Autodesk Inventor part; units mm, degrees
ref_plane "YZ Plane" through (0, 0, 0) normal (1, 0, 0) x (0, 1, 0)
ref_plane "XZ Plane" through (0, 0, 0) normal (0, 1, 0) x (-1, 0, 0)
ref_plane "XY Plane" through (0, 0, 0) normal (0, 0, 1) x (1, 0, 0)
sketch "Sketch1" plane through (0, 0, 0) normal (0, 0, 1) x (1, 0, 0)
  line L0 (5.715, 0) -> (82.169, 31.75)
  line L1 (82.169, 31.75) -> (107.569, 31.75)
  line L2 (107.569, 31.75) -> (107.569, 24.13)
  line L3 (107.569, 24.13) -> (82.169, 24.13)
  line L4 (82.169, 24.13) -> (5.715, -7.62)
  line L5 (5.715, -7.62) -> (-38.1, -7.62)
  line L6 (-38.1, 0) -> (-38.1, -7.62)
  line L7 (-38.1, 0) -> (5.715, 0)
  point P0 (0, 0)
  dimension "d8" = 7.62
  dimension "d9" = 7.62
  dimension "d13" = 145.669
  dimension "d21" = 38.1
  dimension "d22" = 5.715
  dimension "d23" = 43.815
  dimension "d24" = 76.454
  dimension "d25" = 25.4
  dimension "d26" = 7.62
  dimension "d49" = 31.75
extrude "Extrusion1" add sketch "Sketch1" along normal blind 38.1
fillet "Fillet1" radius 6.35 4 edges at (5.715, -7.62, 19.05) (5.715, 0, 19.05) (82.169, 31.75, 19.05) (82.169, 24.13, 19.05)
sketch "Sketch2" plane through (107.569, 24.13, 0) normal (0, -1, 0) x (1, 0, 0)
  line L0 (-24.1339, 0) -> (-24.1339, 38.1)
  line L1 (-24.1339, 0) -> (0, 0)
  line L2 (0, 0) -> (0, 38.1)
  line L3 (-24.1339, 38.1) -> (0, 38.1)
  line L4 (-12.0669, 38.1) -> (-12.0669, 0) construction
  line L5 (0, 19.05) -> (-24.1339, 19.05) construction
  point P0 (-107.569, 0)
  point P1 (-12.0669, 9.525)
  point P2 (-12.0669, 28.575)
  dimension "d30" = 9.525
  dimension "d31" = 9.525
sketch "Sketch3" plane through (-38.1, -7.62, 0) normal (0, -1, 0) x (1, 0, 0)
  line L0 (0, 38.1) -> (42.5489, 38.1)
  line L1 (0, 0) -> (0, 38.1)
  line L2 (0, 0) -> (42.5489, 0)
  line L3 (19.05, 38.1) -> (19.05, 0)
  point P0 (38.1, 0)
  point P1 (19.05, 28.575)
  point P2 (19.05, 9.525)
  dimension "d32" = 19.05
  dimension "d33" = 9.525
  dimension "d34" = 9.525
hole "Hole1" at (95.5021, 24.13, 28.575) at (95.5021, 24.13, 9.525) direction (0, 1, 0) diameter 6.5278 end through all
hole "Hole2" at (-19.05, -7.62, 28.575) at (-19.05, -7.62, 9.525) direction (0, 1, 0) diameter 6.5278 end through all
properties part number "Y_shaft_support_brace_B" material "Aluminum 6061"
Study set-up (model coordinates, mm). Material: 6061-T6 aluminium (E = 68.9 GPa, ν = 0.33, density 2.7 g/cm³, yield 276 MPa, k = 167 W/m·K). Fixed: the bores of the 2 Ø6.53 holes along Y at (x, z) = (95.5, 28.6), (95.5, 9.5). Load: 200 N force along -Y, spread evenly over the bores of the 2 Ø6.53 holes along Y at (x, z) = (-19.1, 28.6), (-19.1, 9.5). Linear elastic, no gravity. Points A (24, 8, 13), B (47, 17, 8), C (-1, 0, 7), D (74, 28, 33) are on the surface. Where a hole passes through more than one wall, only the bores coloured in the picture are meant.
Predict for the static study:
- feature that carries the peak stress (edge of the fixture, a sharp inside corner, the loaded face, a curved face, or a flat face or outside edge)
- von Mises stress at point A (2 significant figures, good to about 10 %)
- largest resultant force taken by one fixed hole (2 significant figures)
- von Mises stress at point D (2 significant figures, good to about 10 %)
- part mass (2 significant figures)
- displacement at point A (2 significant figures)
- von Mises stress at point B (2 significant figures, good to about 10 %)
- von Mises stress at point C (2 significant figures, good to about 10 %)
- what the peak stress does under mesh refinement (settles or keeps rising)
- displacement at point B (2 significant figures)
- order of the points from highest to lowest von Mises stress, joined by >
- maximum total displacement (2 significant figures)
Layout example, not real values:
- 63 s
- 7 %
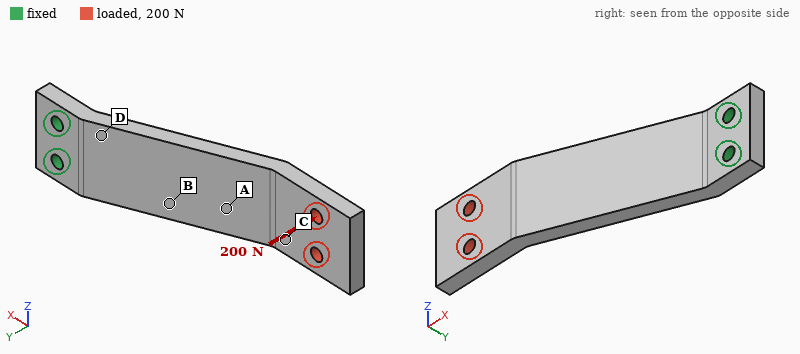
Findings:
- edge of the fixture
- 29 MPa
- 130 N
- 60 MPa
- 110 g
- 0.58 mm
- 43 MPa
- 9.9 MPa
- keeps rising
- 0.27 mm
- D > B > A > C
- 1.6 mm
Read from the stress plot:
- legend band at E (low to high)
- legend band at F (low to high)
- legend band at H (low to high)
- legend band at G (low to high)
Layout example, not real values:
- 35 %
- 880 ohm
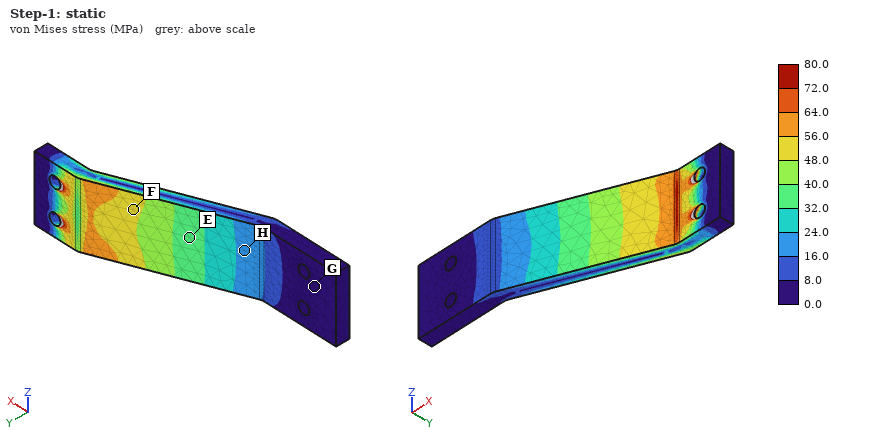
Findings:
- 32.0 to 40.0 MPa
- 48.0 to 56.0 MPa
- 16.0 to 24.0 MPa
- 0.0 to 8.0 MPa
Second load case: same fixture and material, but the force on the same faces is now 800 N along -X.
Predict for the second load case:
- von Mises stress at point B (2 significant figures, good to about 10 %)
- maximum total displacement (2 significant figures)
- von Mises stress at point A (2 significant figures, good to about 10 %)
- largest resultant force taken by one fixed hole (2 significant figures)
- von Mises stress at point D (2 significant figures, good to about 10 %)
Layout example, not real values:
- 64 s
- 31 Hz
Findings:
- 42 MPa
- 1.7 mm
- 18 MPa
- 430 N
- 70 MPa
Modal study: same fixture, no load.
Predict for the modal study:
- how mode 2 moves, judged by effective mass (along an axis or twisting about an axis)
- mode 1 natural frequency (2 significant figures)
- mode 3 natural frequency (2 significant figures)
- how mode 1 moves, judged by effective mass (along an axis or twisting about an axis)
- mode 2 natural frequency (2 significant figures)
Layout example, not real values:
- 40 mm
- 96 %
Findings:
- along Z
- 310 Hz
- 1900 Hz
- along Y
- 1300 Hz
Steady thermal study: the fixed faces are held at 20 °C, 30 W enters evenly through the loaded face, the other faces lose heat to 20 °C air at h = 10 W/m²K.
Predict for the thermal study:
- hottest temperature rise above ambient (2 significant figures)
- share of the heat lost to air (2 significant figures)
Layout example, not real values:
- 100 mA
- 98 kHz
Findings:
- 71 K
- 17 %
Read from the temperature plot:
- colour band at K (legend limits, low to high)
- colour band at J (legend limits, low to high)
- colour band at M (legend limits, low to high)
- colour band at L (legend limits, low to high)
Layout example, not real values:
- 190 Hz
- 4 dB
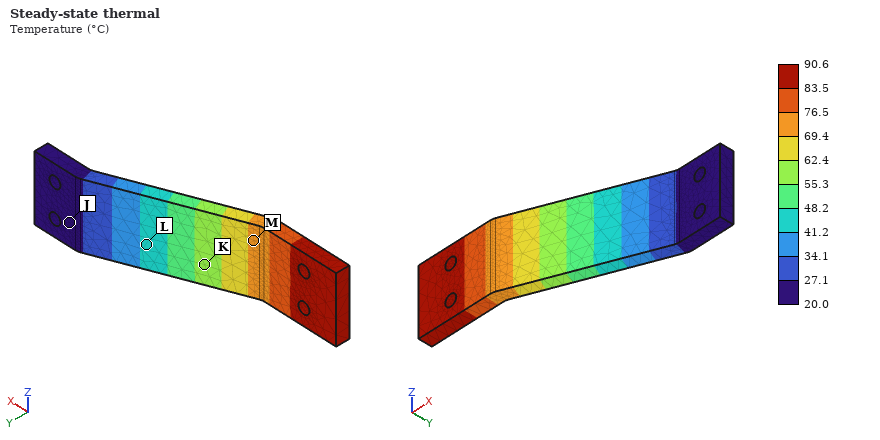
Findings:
- 55.3 to 62.4 °C
- 20.0 to 27.1 °C
- 69.4 to 76.5 °C
- 41.2 to 48.2 °C
